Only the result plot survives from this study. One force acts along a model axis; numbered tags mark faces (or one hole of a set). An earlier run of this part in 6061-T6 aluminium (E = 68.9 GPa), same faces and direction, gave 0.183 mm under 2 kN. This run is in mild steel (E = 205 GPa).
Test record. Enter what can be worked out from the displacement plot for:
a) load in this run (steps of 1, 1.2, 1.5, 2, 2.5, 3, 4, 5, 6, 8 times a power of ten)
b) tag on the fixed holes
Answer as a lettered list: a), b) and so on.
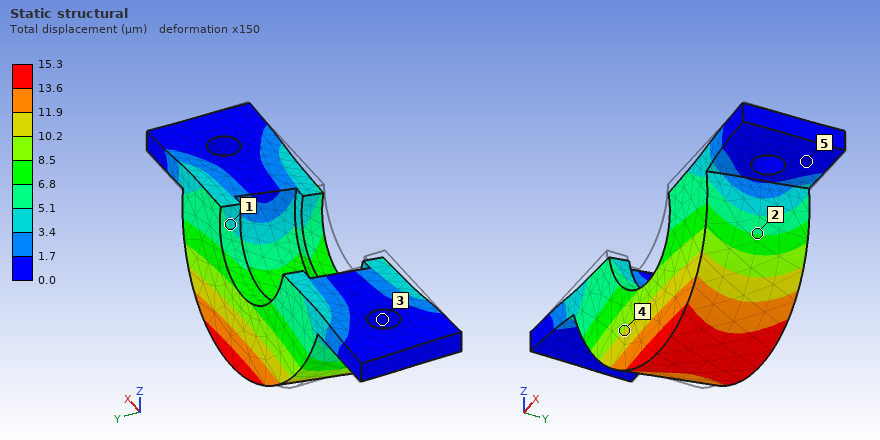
a) 500 N
b) 3
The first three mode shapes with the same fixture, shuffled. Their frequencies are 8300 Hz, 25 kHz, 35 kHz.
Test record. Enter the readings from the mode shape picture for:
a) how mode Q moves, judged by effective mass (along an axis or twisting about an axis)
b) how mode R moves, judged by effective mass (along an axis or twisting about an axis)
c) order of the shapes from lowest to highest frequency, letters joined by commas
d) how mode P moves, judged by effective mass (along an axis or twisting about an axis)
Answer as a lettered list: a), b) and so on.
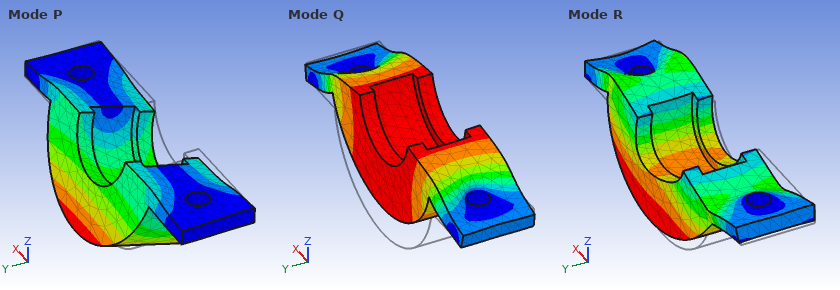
a) along Z
b) along X
c) P, Q, R
d) along Y
